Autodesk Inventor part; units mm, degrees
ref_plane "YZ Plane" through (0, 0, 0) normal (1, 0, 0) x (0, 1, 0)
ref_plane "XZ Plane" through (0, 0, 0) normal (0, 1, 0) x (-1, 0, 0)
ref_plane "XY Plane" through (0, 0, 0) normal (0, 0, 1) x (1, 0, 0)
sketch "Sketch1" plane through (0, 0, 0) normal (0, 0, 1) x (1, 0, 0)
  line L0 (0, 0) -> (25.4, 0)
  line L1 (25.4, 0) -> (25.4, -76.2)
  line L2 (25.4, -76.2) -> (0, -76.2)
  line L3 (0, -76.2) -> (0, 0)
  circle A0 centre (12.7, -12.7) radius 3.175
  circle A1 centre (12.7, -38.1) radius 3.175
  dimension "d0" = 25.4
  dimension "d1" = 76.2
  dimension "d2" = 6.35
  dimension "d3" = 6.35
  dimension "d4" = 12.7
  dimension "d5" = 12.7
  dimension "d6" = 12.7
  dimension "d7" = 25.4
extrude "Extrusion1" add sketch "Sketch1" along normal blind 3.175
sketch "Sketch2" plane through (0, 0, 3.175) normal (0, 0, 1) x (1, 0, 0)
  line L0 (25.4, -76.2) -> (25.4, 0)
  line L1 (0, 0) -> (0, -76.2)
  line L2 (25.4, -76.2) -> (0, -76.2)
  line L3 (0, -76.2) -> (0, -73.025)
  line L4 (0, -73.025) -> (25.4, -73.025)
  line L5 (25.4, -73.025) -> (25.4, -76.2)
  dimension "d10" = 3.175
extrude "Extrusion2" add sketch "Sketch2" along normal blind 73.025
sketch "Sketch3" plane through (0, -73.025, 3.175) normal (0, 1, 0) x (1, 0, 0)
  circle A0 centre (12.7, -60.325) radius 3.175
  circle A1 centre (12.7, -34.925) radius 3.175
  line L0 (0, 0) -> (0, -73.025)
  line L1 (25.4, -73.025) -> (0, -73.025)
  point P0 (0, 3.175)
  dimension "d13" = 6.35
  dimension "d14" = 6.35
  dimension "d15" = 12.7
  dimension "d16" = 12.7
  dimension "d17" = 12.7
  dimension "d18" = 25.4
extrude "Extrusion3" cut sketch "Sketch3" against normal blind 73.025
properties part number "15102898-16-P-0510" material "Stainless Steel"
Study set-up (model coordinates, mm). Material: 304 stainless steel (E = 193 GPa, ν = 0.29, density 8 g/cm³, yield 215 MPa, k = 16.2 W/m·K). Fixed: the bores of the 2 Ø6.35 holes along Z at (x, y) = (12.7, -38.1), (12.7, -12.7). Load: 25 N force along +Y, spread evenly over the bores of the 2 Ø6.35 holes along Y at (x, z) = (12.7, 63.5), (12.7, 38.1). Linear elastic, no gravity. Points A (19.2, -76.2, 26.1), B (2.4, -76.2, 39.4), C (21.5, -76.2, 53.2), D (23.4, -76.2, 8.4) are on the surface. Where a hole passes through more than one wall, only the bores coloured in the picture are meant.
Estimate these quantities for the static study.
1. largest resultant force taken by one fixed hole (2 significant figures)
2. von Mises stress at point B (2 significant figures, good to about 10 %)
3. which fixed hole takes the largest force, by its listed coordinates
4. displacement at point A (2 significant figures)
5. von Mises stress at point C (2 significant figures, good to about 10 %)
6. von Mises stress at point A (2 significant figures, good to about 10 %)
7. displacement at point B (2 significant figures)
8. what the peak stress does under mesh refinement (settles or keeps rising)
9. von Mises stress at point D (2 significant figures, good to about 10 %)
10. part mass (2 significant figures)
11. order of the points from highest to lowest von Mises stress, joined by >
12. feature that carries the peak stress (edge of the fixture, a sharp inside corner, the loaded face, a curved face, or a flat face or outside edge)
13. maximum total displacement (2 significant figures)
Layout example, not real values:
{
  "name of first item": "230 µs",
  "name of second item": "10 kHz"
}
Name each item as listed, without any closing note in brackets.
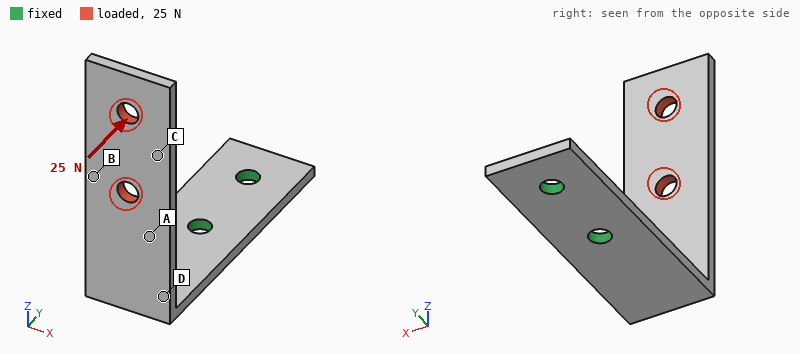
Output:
{
  "largest resultant force taken by one fixed hole": "22 N",
  "von Mises stress at point B": "9.0 MPa",
  "which fixed hole takes the largest force, by its listed coordinates": "(12.7, -38.1)",
  "displacement at point A": "0.12 mm",
  "von Mises stress at point C": "3.2 MPa",
  "von Mises stress at point A": "14 MPa",
  "displacement at point B": "0.18 mm",
  "what the peak stress does under mesh refinement": "keeps rising",
  "von Mises stress at point D": "25 MPa",
  "part mass": "93 g",
  "order of the points from highest to lowest von Mises stress, joined by >": "D > A > B > C",
  "feature that carries the peak stress": "edge of the fixture",
  "maximum total displacement": "0.38 mm"
}
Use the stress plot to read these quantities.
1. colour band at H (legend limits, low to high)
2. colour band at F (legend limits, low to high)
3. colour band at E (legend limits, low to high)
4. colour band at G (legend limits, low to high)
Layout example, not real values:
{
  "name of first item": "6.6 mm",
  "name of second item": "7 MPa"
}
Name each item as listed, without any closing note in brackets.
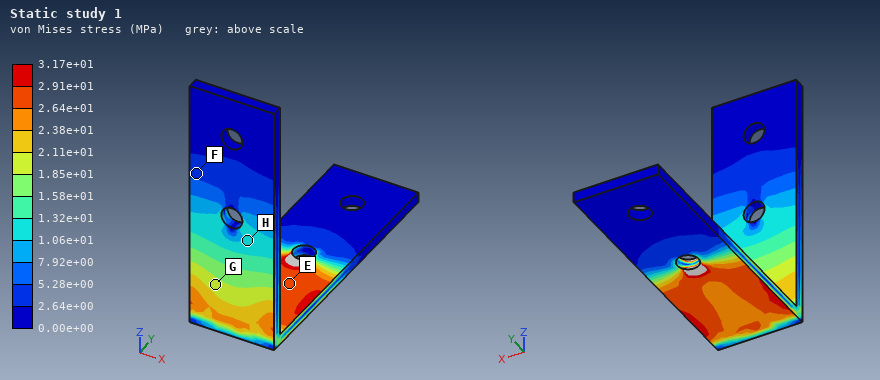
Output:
{
  "colour band at H": "1.06e+01 to 1.32e+01 MPa",
  "colour band at F": "2.64e+00 to 5.28e+00 MPa",
  "colour band at E": "2.64e+01 to 2.91e+01 MPa",
  "colour band at G": "1.85e+01 to 2.11e+01 MPa"
}
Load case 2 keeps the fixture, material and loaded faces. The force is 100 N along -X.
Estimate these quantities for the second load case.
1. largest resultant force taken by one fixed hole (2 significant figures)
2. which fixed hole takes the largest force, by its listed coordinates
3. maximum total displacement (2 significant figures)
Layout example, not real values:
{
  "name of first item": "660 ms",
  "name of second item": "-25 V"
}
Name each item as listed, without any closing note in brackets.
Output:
{
  "largest resultant force taken by one fixed hole": "190 N",
  "which fixed hole takes the largest force, by its listed coordinates": "(12.7, -38.1)",
  "maximum total displacement": "0.62 mm"
}
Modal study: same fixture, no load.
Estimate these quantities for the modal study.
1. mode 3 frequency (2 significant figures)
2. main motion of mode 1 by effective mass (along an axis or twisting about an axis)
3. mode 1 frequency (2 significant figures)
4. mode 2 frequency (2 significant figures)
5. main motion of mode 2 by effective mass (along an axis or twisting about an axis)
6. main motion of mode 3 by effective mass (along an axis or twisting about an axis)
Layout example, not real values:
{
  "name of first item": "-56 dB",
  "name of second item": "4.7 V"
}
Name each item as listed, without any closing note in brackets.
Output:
{
  "mode 3 frequency": "950 Hz",
  "main motion of mode 1 by effective mass": "along Y",
  "mode 1 frequency": "270 Hz",
  "mode 2 frequency": "420 Hz",
  "main motion of mode 2 by effective mass": "along X",
  "main motion of mode 3 by effective mass": "along Z"
}
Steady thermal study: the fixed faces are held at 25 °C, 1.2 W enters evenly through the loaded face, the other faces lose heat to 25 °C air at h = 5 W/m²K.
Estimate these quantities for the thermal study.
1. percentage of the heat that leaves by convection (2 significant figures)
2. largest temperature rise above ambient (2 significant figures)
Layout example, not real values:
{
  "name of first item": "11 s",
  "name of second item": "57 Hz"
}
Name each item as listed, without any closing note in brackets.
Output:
{
  "percentage of the heat that leaves by convection": "59 %",
  "largest temperature rise above ambient": "41 K"
}
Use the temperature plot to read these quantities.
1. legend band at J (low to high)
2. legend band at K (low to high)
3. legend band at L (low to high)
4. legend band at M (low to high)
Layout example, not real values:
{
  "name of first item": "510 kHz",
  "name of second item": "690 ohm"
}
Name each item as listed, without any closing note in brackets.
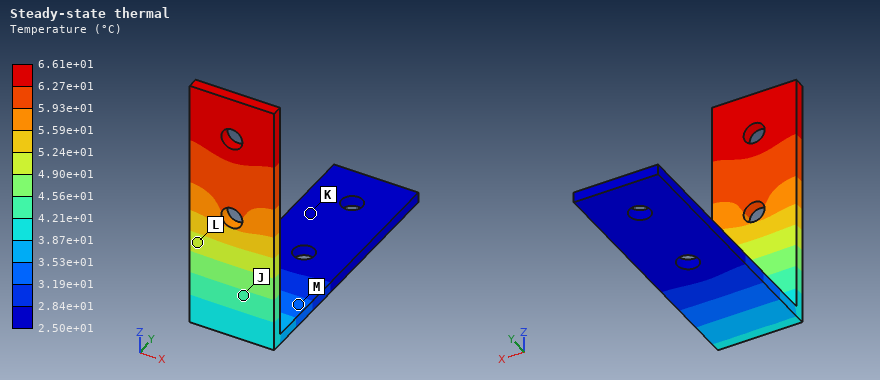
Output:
{
  "legend band at J": "4.21e+01 to 4.56e+01 °C",
  "legend band at K": "2.50e+01 to 2.84e+01 °C",
  "legend band at L": "4.90e+01 to 5.24e+01 °C",
  "legend band at M": "3.19e+01 to 3.53e+01 °C"
}
